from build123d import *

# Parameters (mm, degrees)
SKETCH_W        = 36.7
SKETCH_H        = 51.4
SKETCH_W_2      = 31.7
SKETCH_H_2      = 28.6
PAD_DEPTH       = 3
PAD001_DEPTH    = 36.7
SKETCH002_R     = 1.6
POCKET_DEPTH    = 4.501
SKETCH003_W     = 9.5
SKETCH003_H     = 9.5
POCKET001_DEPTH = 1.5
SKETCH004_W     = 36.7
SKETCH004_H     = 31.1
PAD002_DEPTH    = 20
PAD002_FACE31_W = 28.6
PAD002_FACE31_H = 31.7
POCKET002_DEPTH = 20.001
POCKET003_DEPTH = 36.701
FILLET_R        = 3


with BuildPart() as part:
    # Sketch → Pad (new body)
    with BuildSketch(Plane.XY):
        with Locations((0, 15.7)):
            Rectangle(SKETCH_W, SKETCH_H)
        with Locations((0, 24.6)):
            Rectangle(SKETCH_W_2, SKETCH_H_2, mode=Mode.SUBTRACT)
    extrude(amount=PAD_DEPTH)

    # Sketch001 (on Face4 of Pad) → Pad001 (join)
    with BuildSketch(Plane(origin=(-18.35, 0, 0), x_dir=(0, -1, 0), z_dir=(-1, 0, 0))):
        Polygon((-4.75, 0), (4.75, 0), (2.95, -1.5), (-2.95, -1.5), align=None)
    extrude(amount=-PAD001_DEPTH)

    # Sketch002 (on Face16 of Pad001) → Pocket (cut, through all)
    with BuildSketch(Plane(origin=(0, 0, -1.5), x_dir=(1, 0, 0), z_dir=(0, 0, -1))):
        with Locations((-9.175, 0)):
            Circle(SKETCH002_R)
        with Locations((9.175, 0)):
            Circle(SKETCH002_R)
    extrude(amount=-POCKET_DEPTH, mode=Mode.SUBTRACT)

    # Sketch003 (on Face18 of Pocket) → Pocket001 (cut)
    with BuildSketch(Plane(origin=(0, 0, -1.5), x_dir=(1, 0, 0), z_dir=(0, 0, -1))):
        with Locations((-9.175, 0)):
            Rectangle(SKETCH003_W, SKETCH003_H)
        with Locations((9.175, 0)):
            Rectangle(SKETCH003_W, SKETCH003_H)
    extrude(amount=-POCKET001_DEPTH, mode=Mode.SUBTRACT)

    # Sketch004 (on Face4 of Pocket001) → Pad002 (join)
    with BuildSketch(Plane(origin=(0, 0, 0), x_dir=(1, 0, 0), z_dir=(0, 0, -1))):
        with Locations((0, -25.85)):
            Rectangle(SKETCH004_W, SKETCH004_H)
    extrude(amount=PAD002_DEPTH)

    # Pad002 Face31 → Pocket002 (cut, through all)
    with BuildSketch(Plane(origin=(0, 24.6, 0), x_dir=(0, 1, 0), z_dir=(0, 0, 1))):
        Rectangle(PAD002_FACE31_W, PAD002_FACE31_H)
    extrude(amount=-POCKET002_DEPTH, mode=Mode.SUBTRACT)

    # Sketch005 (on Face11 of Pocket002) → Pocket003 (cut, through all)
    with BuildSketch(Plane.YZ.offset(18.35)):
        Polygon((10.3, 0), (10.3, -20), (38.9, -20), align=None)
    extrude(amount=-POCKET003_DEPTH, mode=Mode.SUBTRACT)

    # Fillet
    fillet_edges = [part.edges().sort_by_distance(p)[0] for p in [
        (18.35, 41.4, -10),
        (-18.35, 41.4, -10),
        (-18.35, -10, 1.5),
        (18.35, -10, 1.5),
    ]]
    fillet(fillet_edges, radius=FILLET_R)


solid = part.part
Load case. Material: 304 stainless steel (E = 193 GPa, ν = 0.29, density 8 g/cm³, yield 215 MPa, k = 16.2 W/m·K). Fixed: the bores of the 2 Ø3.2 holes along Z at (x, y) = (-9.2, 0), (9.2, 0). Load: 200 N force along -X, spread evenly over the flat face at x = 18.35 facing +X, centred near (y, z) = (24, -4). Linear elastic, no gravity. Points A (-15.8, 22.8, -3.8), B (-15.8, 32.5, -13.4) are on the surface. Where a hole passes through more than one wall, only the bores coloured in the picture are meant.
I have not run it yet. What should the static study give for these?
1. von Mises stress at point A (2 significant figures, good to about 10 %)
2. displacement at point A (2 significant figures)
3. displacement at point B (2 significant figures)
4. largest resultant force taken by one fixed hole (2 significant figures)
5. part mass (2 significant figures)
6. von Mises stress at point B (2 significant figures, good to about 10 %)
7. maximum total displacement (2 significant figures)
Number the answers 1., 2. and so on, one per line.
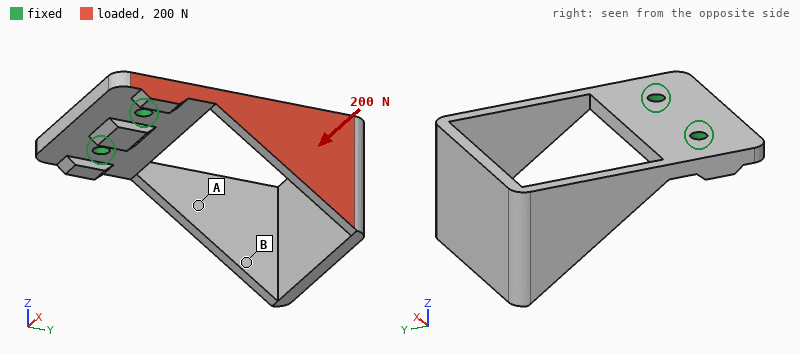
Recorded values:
1. 18 MPa
2. 0.049 mm
3. 0.091 mm
4. 250 N
5. 50 g
6. 39 MPa
7. 0.11 mm
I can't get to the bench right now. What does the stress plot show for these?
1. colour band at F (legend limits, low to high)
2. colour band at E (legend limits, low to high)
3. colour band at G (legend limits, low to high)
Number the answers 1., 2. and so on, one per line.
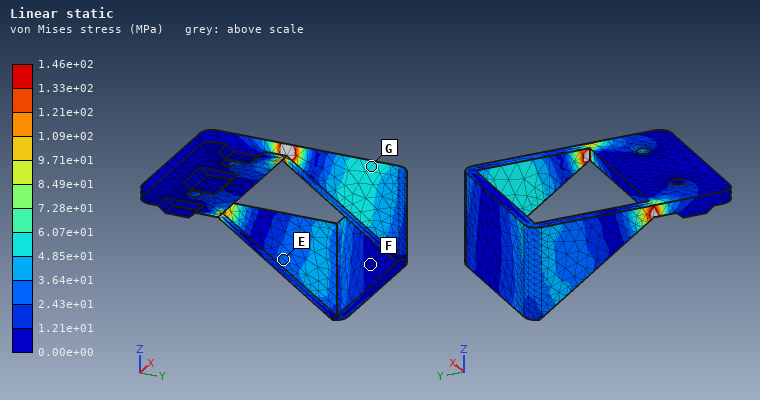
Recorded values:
1. 0.00e+00 to 1.21e+01 MPa
2. 2.43e+01 to 3.64e+01 MPa
3. 4.85e+01 to 6.07e+01 MPa
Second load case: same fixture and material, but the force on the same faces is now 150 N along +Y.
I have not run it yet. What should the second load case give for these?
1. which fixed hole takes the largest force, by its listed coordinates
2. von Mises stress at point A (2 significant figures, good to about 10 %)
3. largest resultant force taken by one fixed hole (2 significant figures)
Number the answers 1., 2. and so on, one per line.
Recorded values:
1. (9.2, 0)
2. 6.9 MPa
3. 210 N
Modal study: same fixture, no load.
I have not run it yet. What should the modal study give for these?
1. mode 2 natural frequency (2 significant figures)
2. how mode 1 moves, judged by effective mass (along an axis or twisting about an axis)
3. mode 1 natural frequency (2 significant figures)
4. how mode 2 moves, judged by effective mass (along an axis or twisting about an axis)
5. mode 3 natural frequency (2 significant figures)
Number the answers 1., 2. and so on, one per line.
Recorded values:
1. 1100 Hz
2. along Z
3. 580 Hz
4. along X
5. 1700 Hz
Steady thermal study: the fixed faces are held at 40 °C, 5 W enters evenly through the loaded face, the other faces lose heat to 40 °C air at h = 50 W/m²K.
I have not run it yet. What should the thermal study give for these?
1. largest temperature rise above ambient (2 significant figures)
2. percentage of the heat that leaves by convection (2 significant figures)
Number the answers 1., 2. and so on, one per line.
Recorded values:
1. 63 K
2. 75 %
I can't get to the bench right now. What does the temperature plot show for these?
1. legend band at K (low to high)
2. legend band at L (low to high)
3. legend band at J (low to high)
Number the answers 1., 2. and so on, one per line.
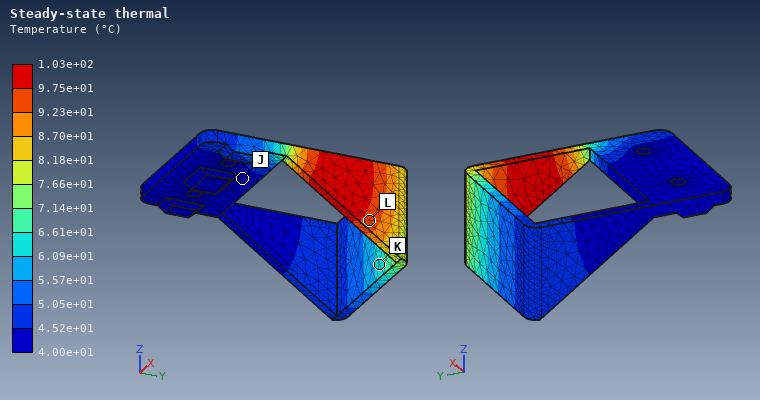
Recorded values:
1. 6.09e+01 to 6.61e+01 °C
2. 9.23e+01 to 9.75e+01 °C
3. 4.00e+01 to 4.52e+01 °C
